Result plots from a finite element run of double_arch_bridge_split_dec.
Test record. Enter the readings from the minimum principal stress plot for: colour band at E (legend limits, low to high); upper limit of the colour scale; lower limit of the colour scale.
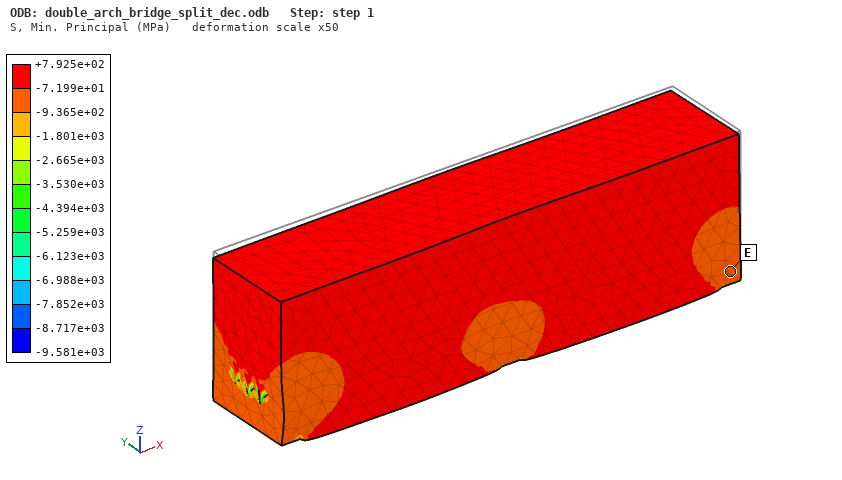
-9.365e+02 to -7.199e+01 MPa
+7.925e+02 MPa
-9.581e+03 MPa
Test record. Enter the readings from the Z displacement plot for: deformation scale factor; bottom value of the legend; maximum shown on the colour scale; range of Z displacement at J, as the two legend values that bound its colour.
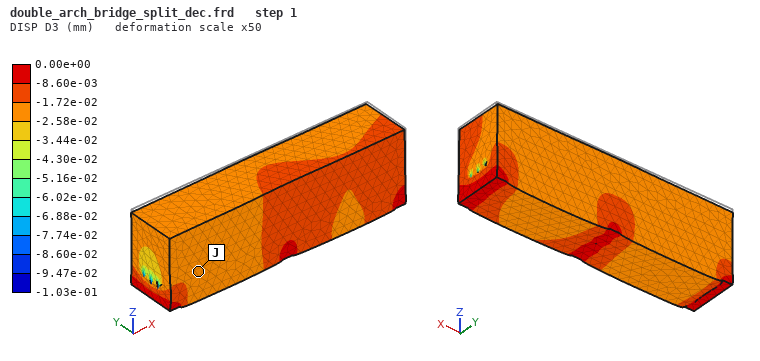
50
-1.03e-01 mm
0.00e+00 mm
-2.58e-02 to -1.72e-02 mm
